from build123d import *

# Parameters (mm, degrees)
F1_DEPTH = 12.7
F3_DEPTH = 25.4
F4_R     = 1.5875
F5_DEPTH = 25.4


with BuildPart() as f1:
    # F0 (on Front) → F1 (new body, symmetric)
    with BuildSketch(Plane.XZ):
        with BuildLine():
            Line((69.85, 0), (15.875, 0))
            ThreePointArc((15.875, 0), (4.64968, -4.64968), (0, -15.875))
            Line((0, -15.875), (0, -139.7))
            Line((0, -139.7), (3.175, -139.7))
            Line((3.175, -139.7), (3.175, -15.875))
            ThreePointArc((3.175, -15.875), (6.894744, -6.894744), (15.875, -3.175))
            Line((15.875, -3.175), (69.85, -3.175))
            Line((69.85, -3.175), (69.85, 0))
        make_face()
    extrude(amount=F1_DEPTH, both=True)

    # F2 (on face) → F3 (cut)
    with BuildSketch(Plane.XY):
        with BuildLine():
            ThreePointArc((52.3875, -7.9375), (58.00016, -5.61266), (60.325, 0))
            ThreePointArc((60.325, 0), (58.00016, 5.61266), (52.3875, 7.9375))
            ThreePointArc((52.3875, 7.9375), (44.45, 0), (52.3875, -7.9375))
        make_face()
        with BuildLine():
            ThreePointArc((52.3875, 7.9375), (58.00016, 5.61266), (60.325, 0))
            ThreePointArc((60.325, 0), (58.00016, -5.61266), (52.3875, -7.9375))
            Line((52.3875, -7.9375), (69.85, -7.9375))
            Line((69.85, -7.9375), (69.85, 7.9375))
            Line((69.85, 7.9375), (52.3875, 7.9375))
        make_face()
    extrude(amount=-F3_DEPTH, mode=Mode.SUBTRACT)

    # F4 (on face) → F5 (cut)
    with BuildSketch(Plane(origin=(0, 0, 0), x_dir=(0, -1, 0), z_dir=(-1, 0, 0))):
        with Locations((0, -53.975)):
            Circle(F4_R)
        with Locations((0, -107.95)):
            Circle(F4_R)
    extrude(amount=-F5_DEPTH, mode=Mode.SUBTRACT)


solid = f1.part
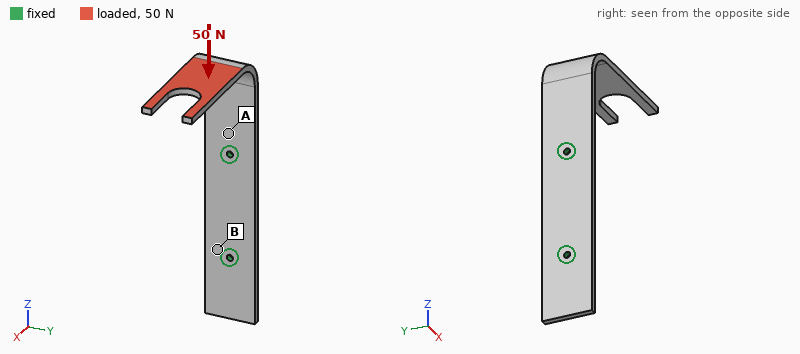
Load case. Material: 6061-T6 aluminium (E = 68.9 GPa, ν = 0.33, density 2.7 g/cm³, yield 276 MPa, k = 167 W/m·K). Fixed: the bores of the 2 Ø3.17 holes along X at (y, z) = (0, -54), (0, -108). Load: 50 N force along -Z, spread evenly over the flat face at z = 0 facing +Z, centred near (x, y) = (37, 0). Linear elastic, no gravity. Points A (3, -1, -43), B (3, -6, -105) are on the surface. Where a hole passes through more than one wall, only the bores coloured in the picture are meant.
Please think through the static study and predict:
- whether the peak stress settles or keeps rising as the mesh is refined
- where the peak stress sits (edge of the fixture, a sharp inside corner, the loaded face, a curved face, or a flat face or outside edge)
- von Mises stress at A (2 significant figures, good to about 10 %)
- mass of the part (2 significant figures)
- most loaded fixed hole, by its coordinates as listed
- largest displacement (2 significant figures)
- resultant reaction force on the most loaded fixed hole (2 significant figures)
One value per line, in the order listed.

keeps rising
edge of the fixture
40 MPa
40 g
(0, -54)
1.7 mm
44 N
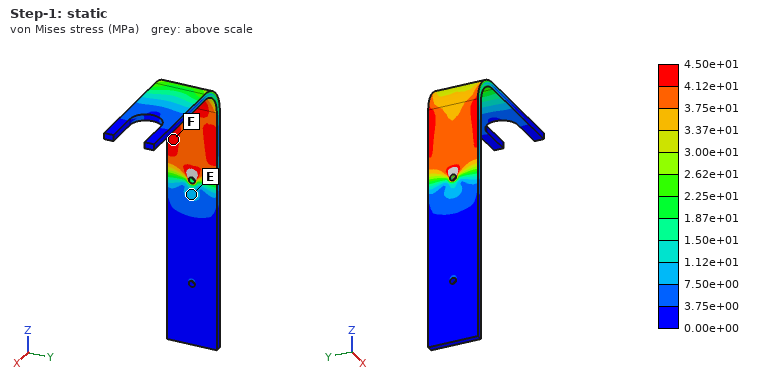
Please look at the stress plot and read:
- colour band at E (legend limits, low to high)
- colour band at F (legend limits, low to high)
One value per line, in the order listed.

7.50e+00 to 1.12e+01 MPa
4.12e+01 to 4.50e+01 MPa
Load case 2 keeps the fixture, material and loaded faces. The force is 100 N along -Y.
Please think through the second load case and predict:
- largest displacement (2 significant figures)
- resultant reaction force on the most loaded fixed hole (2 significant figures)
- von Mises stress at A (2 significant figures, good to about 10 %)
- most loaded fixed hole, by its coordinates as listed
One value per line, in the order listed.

1.8 mm
190 N
78 MPa
(0, -54)
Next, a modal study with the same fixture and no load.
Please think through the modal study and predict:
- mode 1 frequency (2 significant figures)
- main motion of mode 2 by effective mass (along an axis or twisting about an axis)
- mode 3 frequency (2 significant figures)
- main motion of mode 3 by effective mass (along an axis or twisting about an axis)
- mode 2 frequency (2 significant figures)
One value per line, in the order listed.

310 Hz
along Y
910 Hz
along X
500 Hz
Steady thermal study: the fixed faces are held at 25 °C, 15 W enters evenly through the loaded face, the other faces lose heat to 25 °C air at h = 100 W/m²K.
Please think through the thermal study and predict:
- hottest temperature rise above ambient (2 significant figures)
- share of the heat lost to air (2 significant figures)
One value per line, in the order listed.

42 K
71 %
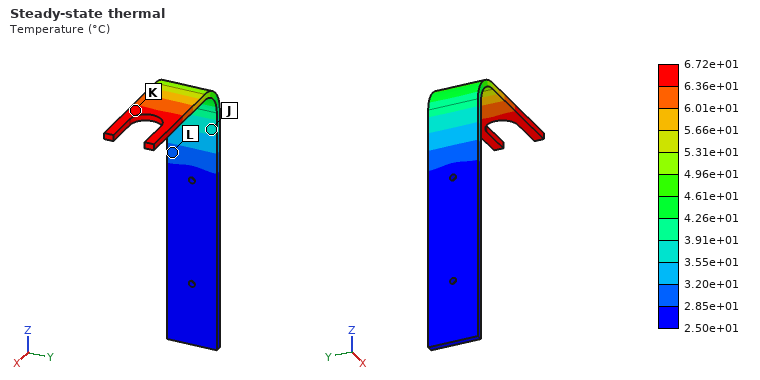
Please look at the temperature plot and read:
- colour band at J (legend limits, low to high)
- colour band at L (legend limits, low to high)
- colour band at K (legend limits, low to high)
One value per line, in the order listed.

3.55e+01 to 3.91e+01 °C
2.85e+01 to 3.20e+01 °C
6.36e+01 to 6.72e+01 °C
